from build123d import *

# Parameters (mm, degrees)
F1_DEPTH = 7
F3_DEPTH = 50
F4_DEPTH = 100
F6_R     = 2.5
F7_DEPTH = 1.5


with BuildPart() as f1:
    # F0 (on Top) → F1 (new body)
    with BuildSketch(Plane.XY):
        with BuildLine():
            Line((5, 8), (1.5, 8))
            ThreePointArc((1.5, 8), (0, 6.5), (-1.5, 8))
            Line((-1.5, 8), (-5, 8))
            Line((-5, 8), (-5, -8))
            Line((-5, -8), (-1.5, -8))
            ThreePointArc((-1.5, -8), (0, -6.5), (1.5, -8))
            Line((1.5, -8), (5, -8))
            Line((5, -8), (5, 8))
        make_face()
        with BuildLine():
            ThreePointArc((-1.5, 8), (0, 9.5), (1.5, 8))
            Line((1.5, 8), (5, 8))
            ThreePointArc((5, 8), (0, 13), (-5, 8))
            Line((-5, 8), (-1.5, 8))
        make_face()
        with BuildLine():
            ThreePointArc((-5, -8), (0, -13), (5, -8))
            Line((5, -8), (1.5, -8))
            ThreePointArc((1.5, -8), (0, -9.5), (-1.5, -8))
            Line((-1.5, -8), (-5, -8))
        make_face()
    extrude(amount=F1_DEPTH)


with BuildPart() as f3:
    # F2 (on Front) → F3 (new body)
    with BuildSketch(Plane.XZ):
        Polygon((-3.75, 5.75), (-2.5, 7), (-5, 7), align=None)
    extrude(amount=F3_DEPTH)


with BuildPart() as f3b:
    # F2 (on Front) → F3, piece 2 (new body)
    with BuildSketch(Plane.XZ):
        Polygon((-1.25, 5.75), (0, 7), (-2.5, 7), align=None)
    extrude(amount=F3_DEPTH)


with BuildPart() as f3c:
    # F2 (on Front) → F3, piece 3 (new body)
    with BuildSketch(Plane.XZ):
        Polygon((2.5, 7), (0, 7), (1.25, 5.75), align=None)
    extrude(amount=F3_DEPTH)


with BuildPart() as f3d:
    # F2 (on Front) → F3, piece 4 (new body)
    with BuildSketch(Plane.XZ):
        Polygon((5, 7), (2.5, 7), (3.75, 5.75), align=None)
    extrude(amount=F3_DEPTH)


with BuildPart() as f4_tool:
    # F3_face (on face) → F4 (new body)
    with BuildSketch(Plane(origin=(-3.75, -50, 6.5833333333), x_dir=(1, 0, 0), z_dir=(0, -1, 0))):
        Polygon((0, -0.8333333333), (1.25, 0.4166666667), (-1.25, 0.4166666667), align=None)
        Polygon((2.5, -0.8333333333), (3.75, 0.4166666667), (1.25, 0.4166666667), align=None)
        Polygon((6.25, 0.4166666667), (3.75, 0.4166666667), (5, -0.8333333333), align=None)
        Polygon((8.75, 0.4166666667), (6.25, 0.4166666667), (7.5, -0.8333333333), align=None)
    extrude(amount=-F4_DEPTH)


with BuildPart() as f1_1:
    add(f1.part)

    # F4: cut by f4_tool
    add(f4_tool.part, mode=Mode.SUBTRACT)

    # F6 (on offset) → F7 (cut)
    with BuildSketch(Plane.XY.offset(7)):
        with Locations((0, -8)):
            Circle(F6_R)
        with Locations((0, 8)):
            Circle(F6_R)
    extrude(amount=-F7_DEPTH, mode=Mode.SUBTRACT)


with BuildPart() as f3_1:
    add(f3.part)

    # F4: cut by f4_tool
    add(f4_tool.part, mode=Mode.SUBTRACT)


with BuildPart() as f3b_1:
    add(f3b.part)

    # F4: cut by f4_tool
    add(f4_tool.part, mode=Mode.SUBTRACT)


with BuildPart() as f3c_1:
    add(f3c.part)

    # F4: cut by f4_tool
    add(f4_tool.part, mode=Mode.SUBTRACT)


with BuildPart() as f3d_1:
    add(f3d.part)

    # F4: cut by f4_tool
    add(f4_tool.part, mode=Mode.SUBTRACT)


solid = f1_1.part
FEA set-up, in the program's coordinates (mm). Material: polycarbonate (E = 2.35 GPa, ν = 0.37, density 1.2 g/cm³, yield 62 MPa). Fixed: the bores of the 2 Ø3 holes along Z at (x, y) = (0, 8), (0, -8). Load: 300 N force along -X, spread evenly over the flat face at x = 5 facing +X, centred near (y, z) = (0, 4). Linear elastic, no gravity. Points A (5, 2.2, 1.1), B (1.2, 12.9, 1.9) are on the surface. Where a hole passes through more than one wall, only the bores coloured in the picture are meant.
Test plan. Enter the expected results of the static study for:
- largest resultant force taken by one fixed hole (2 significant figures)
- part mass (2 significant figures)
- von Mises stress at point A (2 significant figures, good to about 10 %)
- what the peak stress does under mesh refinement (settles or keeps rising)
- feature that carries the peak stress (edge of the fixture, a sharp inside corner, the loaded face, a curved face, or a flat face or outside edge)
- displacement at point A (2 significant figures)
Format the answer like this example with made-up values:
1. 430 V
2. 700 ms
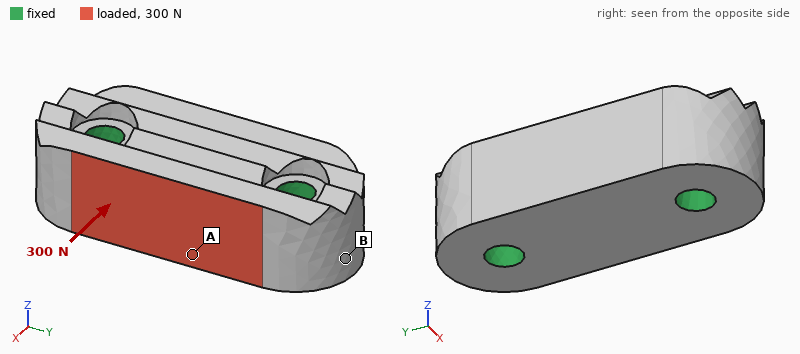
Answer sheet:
1. 150 N
2. 1.7 g
3. 4.0 MPa
4. keeps rising
5. edge of the fixture
6. 17 µm
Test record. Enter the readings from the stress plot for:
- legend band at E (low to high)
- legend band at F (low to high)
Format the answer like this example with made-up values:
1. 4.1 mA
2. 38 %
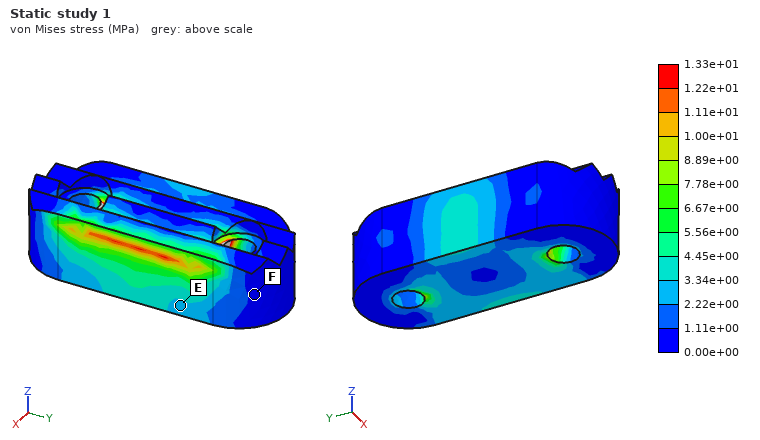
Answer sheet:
1. 2.22e+00 to 3.34e+00 MPa
2. 0.00e+00 to 1.11e+00 MPa
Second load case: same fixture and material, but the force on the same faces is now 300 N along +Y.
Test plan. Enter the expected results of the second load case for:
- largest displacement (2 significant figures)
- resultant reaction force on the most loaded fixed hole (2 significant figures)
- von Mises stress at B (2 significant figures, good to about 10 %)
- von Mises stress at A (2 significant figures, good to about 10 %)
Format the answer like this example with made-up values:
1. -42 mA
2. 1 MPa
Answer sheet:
1. 22 µm
2. 170 N
3. 1.2 MPa
4. 4.7 MPa
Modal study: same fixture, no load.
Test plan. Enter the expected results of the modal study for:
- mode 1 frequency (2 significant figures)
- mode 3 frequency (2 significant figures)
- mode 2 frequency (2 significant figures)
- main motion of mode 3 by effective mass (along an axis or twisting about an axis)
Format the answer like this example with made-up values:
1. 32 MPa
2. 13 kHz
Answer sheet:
1. 19 kHz
2. 21 kHz
3. 19 kHz
4. along X
